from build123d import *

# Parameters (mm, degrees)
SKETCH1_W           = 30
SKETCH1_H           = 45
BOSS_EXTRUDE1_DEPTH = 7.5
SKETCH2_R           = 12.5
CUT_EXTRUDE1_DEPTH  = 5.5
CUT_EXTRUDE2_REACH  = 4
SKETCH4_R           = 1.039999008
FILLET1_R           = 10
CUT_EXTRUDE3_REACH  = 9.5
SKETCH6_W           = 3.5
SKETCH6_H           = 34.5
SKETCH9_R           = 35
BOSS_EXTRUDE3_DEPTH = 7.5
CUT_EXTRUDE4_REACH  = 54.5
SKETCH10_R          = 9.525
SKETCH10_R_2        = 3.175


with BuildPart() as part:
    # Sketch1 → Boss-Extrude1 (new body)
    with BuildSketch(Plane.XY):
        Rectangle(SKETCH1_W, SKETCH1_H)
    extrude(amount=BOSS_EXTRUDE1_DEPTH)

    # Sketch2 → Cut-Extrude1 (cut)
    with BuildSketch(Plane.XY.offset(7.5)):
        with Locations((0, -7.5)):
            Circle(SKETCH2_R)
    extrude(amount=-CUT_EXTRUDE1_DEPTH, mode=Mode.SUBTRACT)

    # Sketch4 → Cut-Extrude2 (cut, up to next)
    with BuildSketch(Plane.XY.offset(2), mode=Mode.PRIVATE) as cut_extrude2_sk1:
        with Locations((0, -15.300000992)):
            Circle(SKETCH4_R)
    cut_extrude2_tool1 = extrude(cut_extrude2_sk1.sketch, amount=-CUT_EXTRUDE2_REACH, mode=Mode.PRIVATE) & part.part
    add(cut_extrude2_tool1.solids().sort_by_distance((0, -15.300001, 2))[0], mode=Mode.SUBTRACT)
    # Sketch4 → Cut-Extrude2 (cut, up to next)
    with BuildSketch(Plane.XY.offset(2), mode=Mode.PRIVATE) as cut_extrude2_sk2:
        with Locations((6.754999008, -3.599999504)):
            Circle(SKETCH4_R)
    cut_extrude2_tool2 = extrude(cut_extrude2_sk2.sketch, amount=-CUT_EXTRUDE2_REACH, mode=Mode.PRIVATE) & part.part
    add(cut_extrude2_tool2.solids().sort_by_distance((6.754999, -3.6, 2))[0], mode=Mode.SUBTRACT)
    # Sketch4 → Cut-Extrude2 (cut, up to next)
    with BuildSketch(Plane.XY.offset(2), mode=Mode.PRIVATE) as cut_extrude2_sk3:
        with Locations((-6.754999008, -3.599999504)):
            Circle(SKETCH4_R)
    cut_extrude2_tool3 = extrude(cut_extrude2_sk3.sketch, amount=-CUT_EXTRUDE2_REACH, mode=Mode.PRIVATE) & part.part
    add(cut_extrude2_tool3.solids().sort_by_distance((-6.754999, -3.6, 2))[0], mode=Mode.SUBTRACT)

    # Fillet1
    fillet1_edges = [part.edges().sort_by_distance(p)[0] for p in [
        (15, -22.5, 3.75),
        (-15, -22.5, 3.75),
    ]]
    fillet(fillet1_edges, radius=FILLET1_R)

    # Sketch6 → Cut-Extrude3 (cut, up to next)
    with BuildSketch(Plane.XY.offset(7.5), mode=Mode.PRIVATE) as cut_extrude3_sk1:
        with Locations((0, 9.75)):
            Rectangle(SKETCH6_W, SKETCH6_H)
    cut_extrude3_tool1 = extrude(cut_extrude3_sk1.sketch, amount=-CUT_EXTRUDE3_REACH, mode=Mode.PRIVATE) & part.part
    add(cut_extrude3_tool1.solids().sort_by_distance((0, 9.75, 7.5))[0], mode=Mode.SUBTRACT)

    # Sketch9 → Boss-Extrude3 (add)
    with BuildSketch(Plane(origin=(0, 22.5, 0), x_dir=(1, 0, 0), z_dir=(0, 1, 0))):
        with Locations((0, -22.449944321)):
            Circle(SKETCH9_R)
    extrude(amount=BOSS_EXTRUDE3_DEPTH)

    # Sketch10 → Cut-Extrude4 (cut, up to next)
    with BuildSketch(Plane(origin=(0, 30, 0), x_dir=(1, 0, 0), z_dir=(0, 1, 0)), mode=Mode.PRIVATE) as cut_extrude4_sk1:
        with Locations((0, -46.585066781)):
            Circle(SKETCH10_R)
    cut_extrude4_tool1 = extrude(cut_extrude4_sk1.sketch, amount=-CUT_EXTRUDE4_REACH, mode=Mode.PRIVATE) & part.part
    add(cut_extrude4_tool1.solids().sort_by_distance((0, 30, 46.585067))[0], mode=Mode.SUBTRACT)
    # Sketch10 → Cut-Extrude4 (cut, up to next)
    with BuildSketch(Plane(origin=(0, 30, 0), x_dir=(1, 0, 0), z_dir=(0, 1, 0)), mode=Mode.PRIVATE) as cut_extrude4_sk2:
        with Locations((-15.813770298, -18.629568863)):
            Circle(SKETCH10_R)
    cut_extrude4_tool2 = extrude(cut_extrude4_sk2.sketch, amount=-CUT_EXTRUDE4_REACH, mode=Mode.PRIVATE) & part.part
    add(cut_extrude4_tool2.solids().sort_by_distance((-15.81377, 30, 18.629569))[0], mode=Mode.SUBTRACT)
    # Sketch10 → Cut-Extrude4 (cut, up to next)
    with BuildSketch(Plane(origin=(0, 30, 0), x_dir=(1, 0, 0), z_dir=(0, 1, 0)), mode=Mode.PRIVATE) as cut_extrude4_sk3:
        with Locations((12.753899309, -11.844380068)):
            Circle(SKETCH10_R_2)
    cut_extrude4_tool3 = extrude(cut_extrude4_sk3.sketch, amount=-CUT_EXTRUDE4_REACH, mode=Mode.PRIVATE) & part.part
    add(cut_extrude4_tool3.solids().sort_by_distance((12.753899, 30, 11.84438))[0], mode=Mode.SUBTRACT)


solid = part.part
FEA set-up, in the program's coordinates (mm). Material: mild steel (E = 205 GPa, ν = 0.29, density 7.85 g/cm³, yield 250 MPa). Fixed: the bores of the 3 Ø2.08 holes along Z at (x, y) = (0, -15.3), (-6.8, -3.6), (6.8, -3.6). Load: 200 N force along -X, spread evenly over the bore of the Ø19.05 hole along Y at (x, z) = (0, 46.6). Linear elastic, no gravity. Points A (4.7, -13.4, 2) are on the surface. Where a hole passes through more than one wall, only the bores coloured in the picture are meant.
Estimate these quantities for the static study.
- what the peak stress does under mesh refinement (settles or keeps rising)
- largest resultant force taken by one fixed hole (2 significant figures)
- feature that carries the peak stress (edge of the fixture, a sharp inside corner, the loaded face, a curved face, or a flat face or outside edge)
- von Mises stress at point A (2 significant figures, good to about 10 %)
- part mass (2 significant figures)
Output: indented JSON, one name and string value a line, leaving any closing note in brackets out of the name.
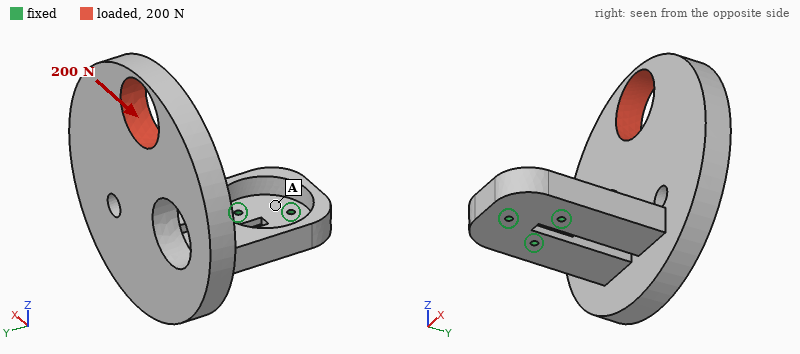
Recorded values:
{
  "what the peak stress does under mesh refinement": "keeps rising",
  "largest resultant force taken by one fixed hole": "570 N",
  "feature that carries the peak stress": "edge of the fixture",
  "von Mises stress at point A": "19 MPa",
  "part mass": "240 g"
}
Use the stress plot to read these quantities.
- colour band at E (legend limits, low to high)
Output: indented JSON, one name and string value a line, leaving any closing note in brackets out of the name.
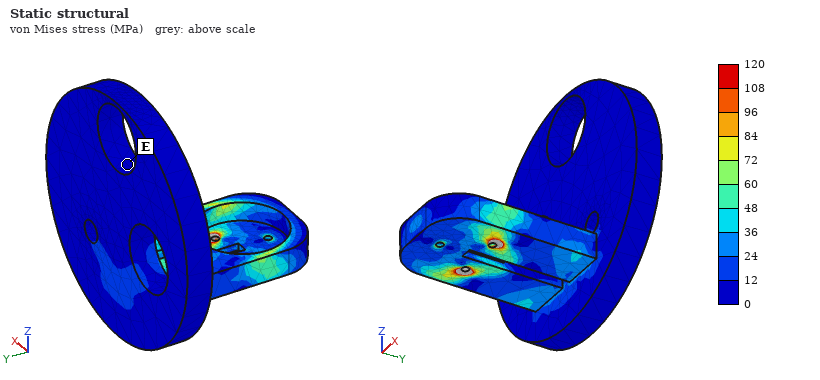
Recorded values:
{
  "colour band at E": "0 to 12 MPa"
}
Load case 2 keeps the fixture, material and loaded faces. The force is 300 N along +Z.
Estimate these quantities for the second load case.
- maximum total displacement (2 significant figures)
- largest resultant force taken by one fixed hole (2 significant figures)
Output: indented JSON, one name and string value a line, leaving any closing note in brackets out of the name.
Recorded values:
{
  "maximum total displacement": "0.17 mm",
  "largest resultant force taken by one fixed hole": "480 N"
}
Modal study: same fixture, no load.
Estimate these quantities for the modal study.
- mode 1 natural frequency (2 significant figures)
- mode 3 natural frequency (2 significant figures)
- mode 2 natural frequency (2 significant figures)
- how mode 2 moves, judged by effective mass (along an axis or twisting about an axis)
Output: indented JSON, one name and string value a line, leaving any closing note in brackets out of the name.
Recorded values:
{
  "mode 1 natural frequency": "510 Hz",
  "mode 3 natural frequency": "2200 Hz",
  "mode 2 natural frequency": "660 Hz",
  "how mode 2 moves, judged by effective mass": "along X"
}
